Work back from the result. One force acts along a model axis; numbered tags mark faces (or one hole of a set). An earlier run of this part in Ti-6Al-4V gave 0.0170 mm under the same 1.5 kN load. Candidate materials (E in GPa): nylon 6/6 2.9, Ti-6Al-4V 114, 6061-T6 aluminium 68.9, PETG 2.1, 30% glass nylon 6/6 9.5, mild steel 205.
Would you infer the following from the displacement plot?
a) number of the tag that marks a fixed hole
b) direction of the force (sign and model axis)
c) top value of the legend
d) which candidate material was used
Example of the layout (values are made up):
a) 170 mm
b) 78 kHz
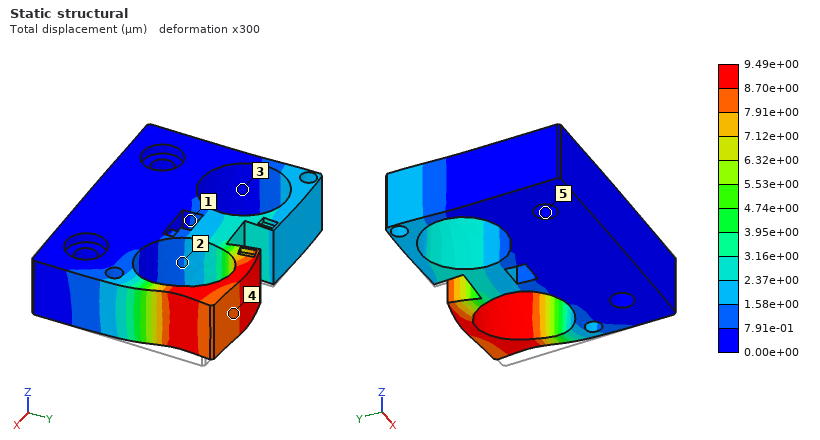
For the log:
a) 5
b) -X
c) 9.49e+00 µm
d) mild steel
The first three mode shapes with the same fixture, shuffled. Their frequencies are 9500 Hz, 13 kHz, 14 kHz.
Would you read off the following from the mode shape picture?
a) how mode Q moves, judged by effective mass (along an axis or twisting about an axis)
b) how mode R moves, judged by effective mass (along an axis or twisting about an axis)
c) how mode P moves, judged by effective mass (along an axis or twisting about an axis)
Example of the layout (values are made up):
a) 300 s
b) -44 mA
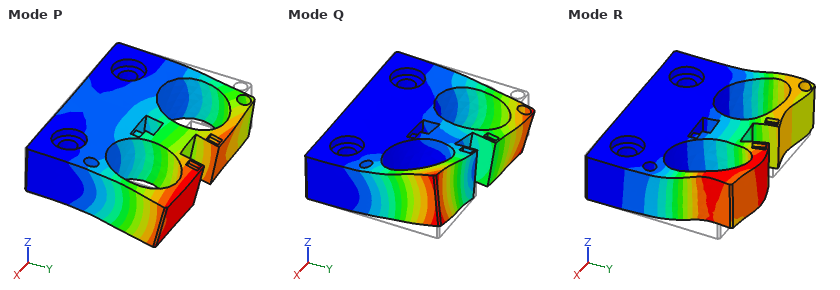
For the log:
a) twisting about Y
b) along X
c) along Z
